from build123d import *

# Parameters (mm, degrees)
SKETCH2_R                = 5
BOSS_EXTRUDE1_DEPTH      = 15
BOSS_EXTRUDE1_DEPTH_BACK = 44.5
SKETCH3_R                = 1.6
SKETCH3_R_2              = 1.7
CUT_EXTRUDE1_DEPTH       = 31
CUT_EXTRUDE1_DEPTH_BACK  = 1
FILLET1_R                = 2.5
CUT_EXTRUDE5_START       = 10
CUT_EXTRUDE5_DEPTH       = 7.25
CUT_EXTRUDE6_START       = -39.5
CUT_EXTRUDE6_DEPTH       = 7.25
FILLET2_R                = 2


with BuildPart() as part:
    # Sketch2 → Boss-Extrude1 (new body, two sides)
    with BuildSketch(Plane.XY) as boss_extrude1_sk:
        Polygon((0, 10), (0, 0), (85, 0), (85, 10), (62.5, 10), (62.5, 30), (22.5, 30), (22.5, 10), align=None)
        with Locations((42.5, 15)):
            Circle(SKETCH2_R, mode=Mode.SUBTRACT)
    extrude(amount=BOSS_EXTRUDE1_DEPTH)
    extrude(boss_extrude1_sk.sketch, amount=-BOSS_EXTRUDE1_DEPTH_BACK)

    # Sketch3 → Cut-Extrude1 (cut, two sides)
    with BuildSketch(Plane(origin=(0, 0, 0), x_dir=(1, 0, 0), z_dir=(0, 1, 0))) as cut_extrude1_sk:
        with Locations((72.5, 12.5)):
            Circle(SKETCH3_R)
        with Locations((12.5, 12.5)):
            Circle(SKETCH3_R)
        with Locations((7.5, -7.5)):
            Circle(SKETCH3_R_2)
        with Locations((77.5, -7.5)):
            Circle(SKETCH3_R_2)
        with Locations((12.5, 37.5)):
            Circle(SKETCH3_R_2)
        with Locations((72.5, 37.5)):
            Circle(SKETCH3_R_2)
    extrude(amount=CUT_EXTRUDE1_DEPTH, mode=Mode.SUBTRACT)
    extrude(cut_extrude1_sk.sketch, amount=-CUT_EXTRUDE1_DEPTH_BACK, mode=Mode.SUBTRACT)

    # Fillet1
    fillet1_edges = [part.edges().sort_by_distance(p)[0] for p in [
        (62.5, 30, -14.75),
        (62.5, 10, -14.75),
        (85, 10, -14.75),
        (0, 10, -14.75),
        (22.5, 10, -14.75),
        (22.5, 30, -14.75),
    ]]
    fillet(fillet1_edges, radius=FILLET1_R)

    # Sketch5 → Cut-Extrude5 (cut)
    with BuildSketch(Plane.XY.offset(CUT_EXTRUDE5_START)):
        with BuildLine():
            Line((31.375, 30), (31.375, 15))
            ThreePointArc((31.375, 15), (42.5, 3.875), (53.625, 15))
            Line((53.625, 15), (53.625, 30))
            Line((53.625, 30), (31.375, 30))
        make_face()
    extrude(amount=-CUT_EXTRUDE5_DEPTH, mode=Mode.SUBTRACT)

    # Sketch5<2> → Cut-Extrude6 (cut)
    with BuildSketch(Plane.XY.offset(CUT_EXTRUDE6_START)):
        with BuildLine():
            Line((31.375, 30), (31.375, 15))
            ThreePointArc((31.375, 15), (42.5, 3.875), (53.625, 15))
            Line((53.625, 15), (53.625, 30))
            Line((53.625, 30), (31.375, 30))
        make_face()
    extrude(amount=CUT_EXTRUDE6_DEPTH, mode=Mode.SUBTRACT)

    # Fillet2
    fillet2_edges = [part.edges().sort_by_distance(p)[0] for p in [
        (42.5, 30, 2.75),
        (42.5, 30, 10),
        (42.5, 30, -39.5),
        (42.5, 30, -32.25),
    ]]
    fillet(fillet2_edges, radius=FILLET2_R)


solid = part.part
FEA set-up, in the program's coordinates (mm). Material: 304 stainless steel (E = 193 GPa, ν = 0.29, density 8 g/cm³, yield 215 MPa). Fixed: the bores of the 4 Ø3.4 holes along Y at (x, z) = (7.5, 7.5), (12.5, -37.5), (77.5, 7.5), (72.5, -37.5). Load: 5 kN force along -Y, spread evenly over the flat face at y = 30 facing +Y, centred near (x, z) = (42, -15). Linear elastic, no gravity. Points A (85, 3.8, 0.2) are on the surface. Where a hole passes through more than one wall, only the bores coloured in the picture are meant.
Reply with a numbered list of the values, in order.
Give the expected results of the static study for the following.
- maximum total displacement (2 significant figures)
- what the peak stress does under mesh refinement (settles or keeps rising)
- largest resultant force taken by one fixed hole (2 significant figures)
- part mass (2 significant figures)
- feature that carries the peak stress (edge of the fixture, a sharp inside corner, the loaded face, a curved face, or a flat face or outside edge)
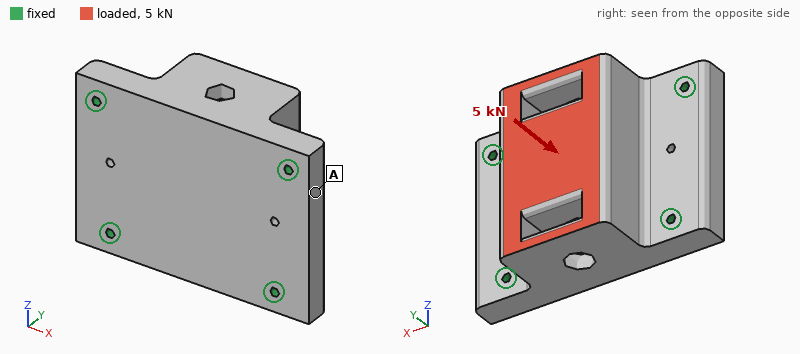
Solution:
1. 5.2 µm
2. keeps rising
3. 1.3 kN
4. 690 g
5. edge of the fixture
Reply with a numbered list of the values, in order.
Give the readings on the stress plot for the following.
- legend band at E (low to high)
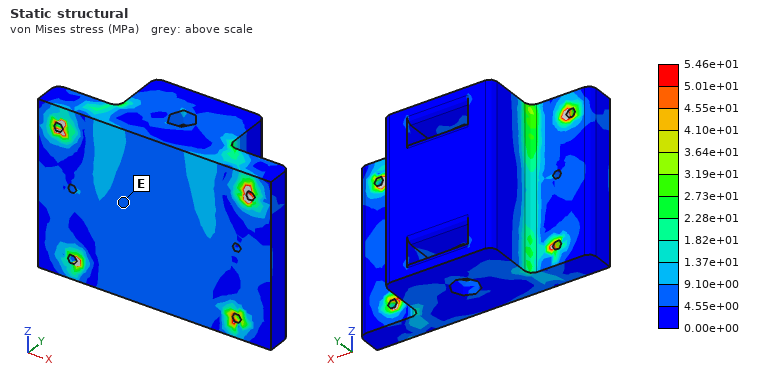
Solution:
1. 4.55e+00 to 9.10e+00 MPa
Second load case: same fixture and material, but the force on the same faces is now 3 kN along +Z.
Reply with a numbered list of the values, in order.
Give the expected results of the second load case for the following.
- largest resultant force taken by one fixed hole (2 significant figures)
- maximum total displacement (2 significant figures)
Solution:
1. 1.3 kN
2. 6.8 µm
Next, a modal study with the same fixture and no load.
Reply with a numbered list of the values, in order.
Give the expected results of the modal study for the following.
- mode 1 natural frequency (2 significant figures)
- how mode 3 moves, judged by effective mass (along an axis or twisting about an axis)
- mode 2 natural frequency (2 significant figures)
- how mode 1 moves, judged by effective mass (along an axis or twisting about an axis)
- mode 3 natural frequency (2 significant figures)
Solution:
1. 7300 Hz
2. along X
3. 9200 Hz
4. along Y
5. 12 kHz
